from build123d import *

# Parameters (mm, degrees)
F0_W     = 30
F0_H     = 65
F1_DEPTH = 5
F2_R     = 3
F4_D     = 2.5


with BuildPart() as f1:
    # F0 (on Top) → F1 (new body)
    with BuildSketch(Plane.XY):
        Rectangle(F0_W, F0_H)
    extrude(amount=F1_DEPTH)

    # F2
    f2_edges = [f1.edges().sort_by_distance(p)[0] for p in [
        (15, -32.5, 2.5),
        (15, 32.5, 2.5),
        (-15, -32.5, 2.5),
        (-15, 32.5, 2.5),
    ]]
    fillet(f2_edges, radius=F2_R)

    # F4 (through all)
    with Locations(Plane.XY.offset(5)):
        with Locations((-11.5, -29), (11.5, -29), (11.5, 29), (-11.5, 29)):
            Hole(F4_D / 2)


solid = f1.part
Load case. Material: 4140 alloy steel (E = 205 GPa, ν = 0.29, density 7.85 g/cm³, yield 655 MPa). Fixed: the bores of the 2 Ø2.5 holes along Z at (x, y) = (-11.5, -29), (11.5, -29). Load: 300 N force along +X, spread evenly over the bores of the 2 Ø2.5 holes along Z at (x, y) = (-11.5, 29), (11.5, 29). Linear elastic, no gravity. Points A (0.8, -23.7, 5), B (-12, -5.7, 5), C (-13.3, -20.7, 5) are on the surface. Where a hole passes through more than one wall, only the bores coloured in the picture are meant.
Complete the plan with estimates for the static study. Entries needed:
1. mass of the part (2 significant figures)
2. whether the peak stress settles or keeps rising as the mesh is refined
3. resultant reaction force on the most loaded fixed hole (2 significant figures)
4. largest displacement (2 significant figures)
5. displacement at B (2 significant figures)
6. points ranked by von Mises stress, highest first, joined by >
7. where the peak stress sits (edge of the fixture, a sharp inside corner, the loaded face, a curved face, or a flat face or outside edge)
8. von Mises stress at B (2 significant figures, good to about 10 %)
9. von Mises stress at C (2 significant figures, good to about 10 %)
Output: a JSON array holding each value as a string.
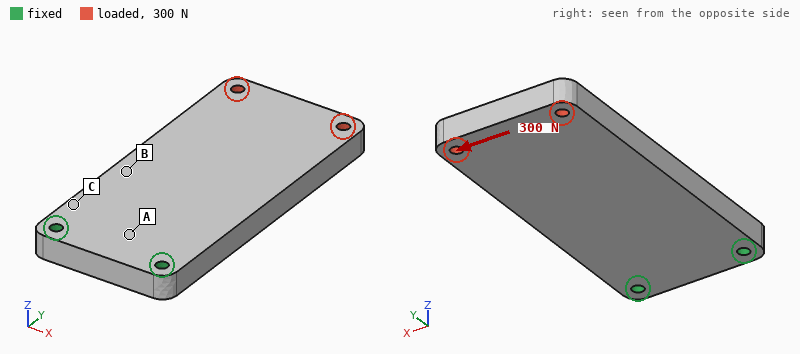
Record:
["75 g", "keeps rising", "750 N", "12 µm", "3.2 µm", "C > B > A", "edge of the fixture", "11 MPa", "18 MPa"]
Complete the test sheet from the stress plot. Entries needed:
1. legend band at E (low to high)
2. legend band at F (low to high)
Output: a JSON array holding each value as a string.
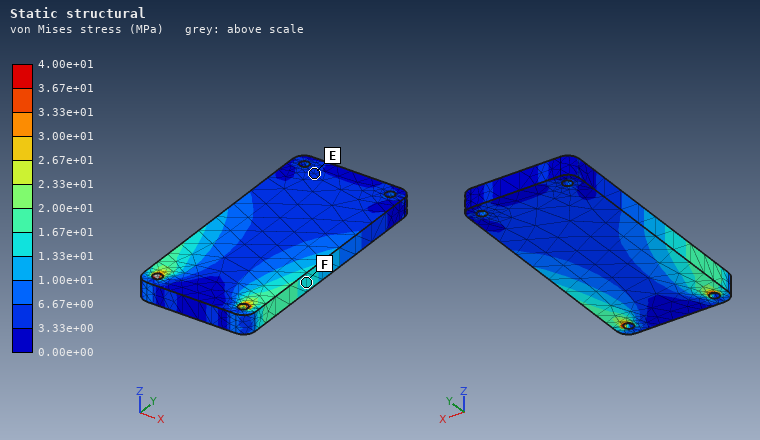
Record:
["3.33e+00 to 6.67e+00 MPa", "1.33e+01 to 1.67e+01 MPa"]
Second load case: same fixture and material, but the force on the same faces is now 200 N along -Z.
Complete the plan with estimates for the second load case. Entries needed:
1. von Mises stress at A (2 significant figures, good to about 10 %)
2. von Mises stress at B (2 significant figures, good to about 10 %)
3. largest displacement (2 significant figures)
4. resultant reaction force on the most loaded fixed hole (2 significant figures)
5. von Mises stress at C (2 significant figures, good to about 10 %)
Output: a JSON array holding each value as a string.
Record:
["58 MPa", "56 MPa", "0.25 mm", "100 N", "89 MPa"]
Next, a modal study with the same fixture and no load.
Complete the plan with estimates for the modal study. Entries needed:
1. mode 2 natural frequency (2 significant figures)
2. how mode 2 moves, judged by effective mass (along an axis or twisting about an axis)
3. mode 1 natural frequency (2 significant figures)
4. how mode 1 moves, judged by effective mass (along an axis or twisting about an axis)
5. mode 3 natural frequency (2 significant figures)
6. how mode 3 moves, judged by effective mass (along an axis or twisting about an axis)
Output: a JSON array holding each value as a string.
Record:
["4600 Hz", "twisting about Y", "1000 Hz", "along Z", "5600 Hz", "along X"]
